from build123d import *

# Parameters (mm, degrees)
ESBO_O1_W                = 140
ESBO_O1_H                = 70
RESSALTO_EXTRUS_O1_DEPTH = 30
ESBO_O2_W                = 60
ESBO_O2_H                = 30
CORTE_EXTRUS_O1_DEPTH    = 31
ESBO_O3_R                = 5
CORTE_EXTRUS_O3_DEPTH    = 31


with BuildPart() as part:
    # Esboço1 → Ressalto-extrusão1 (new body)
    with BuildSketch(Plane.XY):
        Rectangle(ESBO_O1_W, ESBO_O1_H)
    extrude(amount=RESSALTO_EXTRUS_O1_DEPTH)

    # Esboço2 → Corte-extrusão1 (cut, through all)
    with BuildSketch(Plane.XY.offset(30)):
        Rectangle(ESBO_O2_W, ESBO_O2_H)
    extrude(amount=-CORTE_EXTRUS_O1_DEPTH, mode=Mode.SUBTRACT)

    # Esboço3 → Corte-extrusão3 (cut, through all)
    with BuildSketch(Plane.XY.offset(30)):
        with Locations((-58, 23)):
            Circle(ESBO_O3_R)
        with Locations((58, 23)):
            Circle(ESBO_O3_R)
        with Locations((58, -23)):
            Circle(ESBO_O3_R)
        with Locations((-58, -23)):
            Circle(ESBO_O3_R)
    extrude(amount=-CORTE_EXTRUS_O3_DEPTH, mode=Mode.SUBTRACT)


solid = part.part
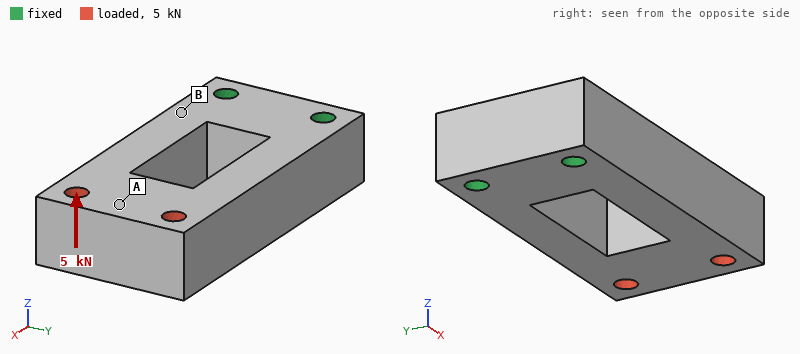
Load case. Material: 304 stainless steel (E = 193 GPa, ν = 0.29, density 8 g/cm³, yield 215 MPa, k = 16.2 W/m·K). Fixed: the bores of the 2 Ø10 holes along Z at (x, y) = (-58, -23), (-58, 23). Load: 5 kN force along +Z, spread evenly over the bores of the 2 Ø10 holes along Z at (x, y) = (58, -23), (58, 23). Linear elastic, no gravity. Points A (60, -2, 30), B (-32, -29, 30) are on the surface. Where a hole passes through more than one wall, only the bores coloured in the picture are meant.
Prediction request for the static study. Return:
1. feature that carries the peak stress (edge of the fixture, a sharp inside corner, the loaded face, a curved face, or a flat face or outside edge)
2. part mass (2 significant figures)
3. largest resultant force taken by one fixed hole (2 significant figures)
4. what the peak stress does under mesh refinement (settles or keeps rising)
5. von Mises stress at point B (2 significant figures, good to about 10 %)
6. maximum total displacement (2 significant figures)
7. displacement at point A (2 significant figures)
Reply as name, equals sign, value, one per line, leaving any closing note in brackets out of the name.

feature that carries the peak stress = edge of the fixture
part mass = 1.8 kg
largest resultant force taken by one fixed hole = 2.5 kN
what the peak stress does under mesh refinement = keeps rising
von Mises stress at point B = 66 MPa
maximum total displacement = 0.16 mm
displacement at point A = 0.14 mm
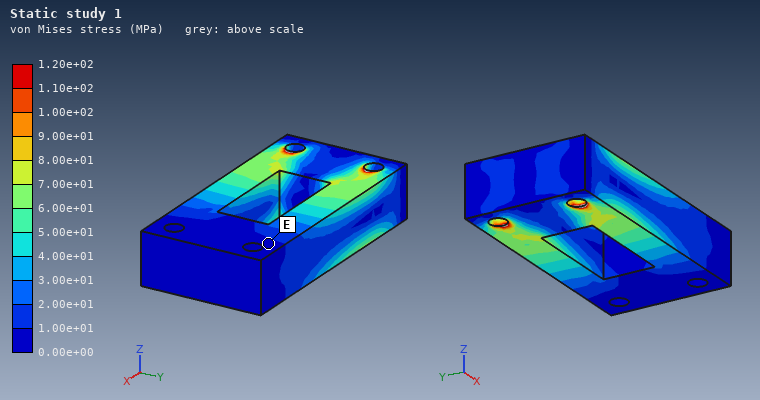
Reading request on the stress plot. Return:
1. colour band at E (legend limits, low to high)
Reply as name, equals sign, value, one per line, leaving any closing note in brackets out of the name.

colour band at E = 0.00e+00 to 1.00e+01 MPa
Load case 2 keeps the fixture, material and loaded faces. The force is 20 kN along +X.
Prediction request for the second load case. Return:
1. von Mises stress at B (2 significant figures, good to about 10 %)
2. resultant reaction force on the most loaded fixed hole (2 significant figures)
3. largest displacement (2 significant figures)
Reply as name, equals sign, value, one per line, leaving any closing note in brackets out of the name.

von Mises stress at B = 15 MPa
resultant reaction force on the most loaded fixed hole = 10 kN
largest displacement = 10 µm
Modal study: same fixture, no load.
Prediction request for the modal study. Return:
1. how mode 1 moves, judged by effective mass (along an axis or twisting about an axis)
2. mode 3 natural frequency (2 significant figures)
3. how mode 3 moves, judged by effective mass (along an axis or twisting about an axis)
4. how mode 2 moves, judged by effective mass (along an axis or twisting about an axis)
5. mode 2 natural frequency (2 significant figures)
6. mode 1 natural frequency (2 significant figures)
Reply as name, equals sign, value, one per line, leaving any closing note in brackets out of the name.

how mode 1 moves, judged by effective mass = along Z
mode 3 natural frequency = 3300 Hz
how mode 3 moves, judged by effective mass = twisting about X
how mode 2 moves, judged by effective mass = along Y
mode 2 natural frequency = 1900 Hz
mode 1 natural frequency = 1200 Hz
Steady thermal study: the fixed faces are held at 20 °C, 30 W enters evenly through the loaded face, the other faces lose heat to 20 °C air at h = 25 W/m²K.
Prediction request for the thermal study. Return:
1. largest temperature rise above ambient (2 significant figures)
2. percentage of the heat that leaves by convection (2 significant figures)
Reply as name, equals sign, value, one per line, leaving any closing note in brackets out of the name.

largest temperature rise above ambient = 66 K
percentage of the heat that leaves by convection = 74 %
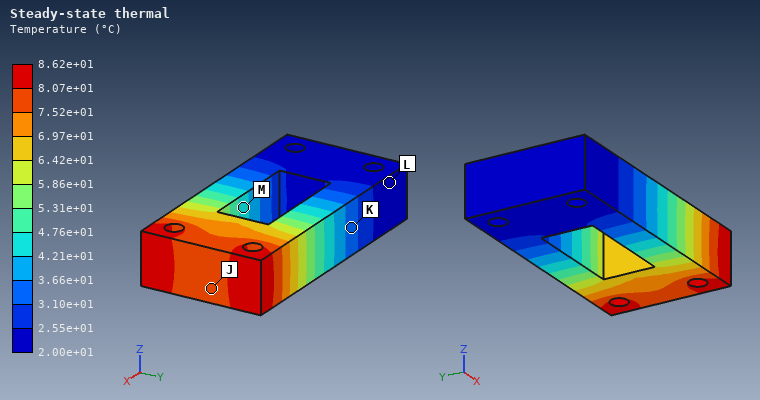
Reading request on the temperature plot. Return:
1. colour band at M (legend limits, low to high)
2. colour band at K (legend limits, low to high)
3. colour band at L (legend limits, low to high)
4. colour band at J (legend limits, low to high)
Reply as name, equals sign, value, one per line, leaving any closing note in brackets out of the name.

colour band at M = 4.21e+01 to 4.76e+01 °C
colour band at K = 3.10e+01 to 3.66e+01 °C
colour band at L = 2.00e+01 to 2.55e+01 °C
colour band at J = 7.52e+01 to 8.07e+01 °C
